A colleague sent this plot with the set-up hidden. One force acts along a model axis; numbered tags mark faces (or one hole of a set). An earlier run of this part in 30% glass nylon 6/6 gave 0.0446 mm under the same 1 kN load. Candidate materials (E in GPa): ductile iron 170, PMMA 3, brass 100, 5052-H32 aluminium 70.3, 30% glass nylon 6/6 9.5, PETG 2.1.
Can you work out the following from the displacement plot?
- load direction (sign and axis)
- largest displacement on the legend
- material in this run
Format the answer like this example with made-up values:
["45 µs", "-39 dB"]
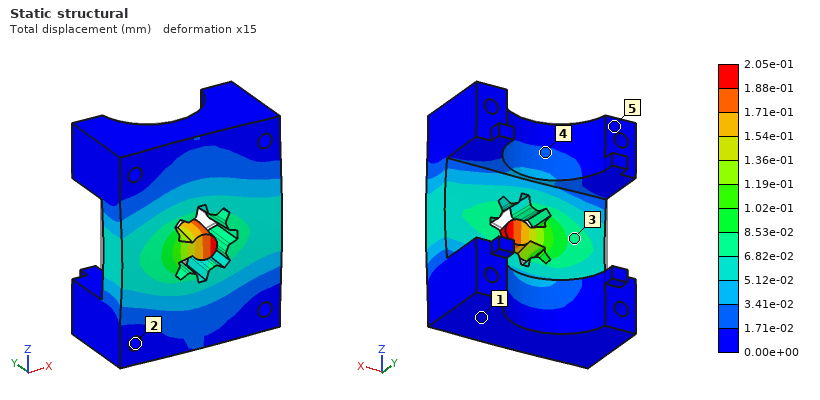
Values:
["-Y", "2.05e-01 mm", "PETG"]
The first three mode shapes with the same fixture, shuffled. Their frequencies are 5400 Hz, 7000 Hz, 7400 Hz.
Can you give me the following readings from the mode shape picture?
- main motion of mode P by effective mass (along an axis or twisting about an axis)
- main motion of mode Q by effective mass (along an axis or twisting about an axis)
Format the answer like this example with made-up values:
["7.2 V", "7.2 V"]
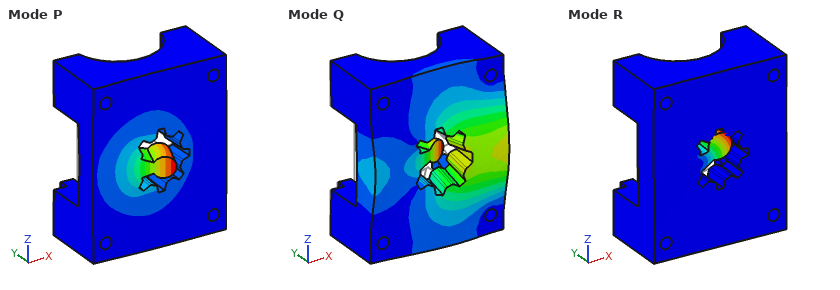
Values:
["along Y", "along Y"]
